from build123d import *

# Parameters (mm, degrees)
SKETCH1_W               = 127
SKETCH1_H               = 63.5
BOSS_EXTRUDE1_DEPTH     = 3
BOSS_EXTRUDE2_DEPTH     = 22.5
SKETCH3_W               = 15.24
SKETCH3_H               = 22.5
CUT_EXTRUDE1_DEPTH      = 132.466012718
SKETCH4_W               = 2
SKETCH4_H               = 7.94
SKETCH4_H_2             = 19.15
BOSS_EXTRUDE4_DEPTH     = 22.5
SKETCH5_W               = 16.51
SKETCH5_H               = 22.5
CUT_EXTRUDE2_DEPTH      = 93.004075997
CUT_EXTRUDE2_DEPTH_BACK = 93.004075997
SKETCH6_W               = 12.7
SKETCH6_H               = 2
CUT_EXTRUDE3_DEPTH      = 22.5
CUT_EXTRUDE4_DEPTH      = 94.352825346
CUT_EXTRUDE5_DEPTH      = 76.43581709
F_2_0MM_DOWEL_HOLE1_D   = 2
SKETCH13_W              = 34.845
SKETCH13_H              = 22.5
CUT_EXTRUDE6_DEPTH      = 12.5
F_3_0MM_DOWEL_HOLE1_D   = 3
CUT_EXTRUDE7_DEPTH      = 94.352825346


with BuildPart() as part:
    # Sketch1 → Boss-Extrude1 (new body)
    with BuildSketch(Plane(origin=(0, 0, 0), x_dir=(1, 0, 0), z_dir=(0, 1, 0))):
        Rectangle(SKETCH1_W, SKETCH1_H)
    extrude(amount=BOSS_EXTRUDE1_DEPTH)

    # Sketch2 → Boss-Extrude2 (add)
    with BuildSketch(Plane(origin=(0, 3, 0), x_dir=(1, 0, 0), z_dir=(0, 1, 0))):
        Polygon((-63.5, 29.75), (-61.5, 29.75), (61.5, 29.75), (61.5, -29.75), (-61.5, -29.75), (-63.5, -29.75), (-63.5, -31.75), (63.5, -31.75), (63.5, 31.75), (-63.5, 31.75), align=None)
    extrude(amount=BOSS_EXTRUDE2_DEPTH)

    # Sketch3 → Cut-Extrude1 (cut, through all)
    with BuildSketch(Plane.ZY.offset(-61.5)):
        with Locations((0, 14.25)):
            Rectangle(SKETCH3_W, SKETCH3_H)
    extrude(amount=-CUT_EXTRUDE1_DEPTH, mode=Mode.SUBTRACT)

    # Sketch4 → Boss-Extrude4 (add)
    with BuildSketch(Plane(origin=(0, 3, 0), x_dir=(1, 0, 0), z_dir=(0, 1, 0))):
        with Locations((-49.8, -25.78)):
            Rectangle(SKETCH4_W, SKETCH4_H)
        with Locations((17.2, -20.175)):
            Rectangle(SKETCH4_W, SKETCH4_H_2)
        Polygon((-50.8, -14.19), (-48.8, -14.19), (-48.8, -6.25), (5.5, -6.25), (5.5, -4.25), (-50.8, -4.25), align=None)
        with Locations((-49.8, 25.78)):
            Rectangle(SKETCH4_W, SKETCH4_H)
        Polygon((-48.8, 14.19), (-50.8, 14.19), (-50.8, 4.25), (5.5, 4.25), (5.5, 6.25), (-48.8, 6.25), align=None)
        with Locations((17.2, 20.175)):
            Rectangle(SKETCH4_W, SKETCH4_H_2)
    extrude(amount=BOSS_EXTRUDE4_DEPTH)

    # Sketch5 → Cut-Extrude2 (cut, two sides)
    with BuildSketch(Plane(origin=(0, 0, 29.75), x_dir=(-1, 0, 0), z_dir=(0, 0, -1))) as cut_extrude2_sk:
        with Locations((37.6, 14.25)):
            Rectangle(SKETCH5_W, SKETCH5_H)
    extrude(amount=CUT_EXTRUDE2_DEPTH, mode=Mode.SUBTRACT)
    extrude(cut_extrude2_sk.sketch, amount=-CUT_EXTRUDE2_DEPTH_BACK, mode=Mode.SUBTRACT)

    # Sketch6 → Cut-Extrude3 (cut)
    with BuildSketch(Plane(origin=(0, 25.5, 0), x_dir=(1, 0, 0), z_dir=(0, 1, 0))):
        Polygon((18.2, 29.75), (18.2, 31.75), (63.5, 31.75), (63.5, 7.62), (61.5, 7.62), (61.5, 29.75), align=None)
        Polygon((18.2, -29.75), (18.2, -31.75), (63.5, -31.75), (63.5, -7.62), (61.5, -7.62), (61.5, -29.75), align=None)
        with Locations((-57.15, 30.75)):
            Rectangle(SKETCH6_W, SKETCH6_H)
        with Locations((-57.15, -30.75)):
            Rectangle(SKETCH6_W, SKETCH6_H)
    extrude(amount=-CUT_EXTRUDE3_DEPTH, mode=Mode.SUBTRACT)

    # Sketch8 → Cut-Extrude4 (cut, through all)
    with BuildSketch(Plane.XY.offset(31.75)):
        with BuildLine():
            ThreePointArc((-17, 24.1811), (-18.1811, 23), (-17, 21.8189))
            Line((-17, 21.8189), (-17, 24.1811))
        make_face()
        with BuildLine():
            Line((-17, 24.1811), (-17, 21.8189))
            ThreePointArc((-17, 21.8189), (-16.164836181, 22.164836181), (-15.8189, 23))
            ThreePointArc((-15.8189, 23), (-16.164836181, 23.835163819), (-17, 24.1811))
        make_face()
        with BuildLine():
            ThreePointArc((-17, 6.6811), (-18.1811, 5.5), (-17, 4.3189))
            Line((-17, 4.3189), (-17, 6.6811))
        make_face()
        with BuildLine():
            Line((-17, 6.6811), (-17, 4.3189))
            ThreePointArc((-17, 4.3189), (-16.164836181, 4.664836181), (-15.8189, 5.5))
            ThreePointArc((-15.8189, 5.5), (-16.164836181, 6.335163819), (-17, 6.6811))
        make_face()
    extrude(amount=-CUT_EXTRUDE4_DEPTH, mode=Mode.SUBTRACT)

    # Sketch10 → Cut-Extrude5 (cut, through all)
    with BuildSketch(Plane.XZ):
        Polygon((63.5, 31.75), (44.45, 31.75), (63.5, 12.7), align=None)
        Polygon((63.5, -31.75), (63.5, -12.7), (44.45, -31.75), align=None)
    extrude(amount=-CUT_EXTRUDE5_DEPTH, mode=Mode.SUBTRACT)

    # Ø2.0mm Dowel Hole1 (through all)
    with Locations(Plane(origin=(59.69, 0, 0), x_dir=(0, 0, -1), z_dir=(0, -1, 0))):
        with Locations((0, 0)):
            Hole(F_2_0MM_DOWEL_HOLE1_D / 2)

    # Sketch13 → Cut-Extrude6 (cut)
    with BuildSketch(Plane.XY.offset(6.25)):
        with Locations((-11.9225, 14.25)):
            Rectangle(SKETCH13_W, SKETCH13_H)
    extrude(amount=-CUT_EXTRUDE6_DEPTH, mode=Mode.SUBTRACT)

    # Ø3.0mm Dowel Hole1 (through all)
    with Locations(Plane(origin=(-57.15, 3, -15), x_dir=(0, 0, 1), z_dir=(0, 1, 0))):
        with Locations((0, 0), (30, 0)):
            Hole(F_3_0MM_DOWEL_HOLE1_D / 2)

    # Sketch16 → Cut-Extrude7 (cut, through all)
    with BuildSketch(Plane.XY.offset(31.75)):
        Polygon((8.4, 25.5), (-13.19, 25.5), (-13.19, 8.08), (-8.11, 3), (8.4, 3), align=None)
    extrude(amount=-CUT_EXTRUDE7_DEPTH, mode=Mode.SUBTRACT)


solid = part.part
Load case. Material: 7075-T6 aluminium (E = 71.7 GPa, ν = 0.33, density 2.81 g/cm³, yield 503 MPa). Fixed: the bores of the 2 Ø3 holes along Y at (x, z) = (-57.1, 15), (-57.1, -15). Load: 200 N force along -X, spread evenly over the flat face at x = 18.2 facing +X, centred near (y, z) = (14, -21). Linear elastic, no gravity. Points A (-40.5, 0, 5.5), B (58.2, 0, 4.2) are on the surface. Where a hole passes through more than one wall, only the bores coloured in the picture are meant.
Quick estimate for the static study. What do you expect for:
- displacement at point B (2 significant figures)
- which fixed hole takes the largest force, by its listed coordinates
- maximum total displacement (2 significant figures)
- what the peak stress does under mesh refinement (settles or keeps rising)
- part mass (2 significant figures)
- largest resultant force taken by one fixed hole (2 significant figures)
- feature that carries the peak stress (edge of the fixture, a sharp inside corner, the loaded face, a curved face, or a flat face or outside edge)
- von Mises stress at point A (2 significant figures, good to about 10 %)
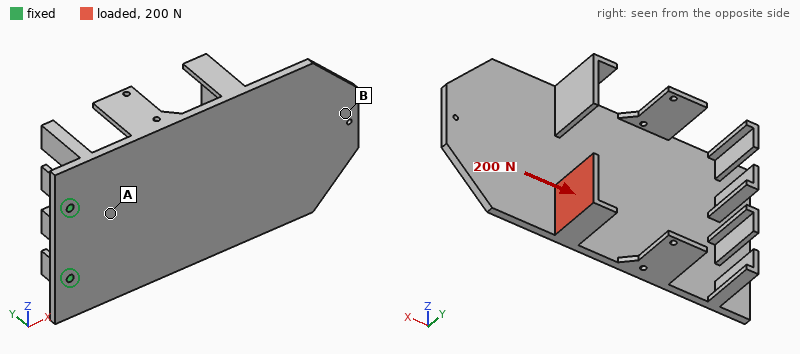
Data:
1.3 mm
(-57.1, -15)
1.5 mm
keeps rising
83 g
230 N
edge of the fixture
23 MPa
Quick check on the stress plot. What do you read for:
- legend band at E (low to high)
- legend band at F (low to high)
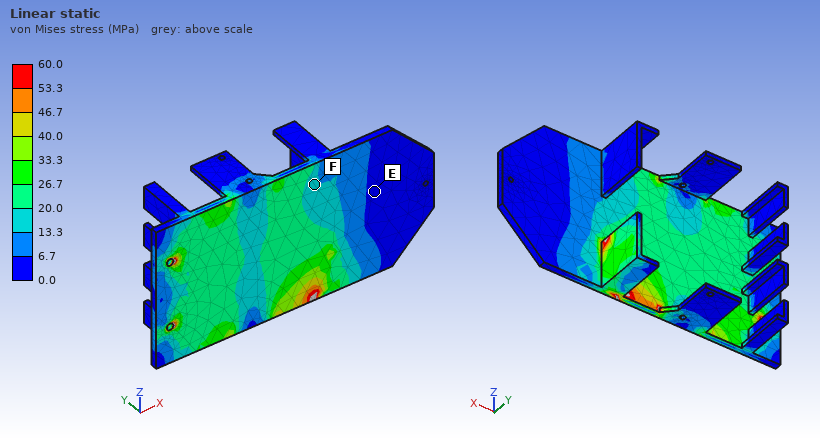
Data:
0.0 to 6.7 MPa
13.3 to 20.0 MPa
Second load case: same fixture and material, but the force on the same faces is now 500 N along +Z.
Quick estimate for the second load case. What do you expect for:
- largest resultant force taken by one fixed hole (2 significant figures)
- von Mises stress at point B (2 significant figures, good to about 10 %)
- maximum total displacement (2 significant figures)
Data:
1.2 kN
12 MPa
1.1 mm
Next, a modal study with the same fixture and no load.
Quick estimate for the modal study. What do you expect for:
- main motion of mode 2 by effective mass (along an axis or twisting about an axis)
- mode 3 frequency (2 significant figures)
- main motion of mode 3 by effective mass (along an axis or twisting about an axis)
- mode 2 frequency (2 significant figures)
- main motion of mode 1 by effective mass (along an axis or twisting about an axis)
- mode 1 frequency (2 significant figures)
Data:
twisting about X
1000 Hz
along Y
600 Hz
along Y
170 Hz
